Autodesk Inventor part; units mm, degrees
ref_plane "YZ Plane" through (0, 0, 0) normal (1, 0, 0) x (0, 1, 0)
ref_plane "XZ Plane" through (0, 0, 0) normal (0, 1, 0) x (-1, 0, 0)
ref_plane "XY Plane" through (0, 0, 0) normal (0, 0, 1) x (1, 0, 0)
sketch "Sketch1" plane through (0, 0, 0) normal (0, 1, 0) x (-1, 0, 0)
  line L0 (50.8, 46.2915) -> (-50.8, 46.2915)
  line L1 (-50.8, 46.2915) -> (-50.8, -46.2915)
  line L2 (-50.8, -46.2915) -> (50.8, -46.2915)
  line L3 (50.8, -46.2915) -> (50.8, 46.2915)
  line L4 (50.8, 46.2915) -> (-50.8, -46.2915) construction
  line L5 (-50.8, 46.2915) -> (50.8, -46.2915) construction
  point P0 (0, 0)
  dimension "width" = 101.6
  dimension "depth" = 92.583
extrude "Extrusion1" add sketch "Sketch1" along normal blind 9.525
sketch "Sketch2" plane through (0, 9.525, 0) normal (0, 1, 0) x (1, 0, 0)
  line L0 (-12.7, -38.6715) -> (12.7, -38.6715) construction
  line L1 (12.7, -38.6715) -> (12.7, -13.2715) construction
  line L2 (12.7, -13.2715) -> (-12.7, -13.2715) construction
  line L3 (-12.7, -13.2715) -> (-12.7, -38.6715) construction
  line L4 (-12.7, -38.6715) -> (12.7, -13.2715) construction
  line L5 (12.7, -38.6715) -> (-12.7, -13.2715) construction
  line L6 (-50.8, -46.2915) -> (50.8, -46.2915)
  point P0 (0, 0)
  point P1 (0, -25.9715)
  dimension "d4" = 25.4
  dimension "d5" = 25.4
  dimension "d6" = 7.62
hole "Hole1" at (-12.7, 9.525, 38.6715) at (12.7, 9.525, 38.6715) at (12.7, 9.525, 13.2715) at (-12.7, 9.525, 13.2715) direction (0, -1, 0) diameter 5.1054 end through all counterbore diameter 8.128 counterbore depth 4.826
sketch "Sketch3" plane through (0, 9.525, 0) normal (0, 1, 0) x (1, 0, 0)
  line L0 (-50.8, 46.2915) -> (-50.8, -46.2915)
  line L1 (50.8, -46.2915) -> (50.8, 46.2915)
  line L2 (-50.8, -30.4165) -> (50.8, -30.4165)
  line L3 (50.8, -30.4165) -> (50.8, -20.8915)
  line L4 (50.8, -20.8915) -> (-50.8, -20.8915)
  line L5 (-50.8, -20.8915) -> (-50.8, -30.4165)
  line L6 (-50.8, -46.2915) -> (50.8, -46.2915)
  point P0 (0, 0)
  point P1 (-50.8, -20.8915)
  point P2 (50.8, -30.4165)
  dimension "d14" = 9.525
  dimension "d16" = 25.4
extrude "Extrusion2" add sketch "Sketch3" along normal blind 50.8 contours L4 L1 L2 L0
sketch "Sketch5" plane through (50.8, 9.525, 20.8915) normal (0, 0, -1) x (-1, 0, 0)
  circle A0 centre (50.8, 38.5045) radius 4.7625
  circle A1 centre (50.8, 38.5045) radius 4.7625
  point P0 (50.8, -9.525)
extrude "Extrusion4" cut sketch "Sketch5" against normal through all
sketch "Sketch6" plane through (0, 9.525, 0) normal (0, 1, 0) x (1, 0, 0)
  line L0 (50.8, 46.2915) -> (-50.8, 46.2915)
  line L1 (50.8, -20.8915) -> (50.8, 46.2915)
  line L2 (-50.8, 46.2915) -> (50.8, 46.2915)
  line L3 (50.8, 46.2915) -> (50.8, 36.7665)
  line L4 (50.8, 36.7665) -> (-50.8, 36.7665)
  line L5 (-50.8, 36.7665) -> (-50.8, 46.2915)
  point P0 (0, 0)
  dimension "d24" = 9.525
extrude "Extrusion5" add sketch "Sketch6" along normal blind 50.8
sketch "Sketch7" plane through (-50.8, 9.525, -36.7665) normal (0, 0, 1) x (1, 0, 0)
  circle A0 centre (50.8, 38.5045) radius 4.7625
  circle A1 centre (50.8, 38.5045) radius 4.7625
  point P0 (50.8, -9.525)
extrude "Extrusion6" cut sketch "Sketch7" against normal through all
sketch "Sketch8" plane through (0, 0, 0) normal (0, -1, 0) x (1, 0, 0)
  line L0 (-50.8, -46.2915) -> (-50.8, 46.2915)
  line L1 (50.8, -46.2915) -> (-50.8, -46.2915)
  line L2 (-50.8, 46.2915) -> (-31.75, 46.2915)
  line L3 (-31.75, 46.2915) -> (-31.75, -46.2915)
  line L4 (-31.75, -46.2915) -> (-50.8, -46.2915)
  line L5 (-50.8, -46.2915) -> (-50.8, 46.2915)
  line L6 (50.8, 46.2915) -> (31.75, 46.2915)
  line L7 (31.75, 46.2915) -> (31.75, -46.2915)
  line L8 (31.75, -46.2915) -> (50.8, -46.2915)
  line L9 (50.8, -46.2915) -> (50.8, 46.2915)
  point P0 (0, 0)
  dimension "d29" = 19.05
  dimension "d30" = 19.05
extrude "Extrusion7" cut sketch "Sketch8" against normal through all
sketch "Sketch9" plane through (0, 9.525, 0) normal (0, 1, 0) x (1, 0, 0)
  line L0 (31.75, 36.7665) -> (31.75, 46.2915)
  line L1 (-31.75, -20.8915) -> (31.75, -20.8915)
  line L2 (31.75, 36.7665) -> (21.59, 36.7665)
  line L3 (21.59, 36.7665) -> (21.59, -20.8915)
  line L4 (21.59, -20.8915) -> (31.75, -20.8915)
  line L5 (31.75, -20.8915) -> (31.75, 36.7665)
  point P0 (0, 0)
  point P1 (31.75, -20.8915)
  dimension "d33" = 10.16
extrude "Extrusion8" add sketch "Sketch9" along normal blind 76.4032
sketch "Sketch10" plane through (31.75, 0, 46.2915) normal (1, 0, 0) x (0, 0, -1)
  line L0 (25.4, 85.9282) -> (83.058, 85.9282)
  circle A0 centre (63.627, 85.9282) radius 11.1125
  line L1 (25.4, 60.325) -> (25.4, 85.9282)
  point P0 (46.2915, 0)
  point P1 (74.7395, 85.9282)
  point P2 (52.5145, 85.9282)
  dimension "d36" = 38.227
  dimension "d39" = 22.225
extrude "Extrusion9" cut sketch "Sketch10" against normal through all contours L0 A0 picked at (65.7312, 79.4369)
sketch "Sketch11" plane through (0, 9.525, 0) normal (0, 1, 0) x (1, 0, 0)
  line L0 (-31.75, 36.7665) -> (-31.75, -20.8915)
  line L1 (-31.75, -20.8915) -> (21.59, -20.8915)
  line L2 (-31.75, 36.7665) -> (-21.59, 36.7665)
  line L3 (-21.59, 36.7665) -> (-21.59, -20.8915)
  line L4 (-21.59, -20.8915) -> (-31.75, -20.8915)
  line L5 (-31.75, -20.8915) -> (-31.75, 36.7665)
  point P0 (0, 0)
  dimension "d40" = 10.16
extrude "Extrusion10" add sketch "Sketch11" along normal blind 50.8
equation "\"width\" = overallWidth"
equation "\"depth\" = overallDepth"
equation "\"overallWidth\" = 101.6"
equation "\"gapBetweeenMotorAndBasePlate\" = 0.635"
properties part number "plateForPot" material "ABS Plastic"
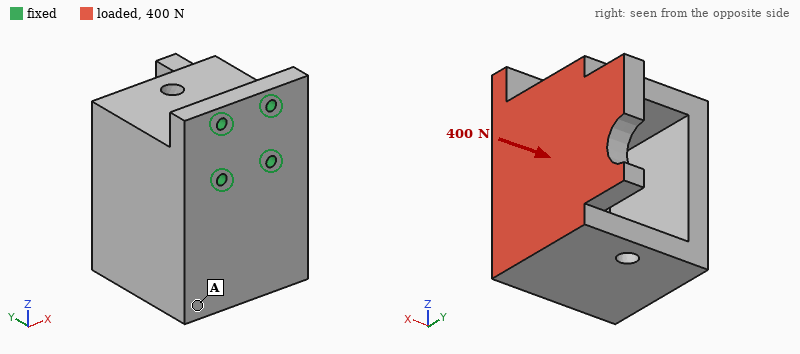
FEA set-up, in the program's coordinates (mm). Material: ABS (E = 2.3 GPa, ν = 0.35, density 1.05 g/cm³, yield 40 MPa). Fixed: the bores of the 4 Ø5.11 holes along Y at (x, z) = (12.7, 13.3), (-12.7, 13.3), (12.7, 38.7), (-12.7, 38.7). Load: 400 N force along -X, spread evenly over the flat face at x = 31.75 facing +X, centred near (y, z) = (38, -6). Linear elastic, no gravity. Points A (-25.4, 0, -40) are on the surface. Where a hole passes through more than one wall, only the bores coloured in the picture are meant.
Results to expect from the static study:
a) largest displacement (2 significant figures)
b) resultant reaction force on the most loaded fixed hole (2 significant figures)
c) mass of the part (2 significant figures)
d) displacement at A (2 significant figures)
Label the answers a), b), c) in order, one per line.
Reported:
a) 0.50 mm
b) 400 N
c) 200 g
d) 0.11 mm
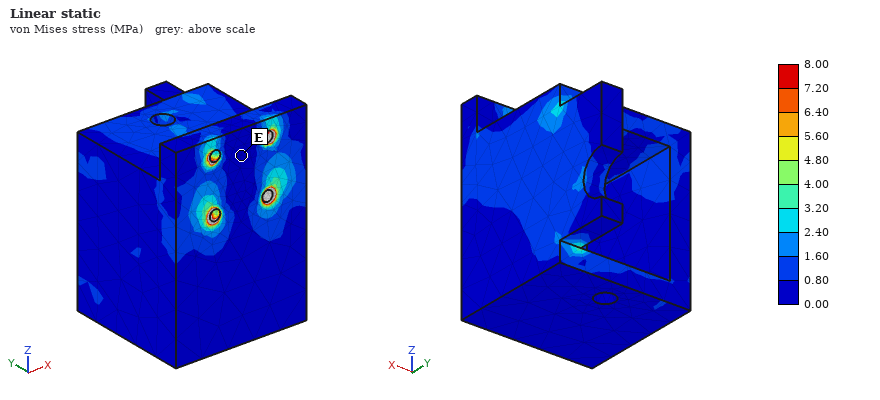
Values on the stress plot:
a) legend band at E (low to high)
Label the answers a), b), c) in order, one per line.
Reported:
a) 0.00 to 0.80 MPa
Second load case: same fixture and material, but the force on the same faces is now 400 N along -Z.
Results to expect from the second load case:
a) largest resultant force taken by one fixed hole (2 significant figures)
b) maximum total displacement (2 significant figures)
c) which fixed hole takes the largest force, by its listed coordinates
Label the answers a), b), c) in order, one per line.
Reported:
a) 440 N
b) 0.52 mm
c) (12.7, 38.7)
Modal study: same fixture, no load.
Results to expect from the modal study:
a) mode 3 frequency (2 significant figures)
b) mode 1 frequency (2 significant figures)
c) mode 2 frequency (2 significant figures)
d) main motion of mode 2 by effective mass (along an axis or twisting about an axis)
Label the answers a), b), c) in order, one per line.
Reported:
a) 1100 Hz
b) 400 Hz
c) 550 Hz
d) along X
